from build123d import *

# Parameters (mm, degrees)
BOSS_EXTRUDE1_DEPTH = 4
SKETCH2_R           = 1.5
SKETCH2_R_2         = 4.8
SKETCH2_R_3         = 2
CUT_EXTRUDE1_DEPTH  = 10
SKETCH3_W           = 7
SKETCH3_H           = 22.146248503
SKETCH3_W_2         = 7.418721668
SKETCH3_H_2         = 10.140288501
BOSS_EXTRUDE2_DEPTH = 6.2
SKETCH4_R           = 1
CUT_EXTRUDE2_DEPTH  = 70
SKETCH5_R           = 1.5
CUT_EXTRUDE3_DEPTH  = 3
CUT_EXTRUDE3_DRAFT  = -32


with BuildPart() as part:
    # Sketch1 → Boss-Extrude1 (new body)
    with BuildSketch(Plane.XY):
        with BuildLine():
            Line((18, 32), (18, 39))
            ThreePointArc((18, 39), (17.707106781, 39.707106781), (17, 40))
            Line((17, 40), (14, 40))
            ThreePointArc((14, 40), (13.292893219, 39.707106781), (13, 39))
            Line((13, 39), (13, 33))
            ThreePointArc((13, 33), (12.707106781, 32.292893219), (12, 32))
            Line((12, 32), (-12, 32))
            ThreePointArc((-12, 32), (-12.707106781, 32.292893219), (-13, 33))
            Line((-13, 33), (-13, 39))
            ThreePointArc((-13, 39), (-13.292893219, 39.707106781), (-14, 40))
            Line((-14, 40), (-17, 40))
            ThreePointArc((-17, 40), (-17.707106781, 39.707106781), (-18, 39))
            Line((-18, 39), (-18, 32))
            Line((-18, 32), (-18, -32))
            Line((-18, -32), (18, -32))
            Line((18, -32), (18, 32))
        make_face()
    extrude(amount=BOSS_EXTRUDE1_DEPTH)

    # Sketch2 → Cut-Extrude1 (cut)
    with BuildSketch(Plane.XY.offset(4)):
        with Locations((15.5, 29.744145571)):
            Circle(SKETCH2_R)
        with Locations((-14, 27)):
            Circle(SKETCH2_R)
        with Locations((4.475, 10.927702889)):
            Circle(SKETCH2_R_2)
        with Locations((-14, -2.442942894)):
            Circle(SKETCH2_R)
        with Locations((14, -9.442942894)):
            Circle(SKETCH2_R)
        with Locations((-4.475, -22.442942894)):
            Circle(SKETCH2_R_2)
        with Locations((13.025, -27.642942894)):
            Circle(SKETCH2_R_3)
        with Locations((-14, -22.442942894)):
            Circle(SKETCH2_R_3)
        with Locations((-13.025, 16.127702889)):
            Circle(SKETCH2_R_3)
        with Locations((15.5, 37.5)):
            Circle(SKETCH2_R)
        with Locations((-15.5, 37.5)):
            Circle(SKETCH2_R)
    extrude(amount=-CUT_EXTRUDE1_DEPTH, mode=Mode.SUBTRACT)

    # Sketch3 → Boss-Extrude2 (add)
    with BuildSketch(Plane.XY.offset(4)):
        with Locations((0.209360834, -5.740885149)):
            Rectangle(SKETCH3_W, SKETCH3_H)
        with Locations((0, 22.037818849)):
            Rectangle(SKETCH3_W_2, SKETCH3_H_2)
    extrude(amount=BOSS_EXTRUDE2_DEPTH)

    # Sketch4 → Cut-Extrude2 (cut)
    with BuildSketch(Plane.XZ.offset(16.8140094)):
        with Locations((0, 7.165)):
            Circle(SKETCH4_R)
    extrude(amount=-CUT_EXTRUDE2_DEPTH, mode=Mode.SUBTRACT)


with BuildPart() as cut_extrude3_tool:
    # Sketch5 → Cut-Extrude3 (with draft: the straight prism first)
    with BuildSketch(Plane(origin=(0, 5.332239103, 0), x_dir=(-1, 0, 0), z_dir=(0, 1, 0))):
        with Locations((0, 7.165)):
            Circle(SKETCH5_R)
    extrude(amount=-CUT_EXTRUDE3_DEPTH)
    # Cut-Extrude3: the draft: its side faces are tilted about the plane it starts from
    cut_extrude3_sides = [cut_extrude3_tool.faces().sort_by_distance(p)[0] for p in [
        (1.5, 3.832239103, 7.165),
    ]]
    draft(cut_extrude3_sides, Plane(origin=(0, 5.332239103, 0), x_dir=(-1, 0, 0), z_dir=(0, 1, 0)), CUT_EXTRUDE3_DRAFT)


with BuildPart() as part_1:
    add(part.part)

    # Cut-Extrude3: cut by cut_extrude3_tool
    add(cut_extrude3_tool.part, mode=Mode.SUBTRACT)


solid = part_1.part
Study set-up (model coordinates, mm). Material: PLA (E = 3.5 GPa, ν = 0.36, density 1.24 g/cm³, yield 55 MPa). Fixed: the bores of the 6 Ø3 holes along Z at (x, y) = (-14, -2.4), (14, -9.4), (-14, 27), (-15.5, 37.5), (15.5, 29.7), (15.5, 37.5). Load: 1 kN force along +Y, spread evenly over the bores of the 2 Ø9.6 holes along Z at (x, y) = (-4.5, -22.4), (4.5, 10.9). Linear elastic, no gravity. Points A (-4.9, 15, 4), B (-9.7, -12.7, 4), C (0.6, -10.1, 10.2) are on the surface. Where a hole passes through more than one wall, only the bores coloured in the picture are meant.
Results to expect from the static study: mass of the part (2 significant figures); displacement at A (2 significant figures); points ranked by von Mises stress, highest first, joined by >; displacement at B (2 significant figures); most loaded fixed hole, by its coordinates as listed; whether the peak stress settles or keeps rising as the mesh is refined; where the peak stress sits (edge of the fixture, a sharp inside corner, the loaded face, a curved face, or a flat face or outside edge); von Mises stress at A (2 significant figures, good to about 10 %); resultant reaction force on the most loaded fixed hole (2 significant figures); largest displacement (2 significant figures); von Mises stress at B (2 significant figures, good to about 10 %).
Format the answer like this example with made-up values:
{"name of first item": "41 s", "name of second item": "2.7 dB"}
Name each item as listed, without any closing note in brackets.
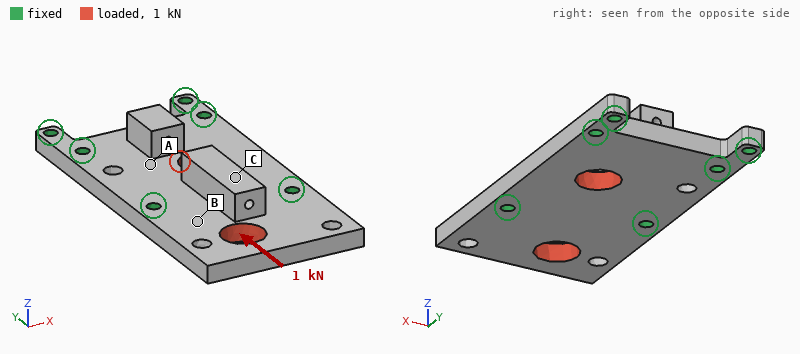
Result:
{"mass of the part": "12 g", "displacement at A": "16 µm", "points ranked by von Mises stress, highest first, joined by >": "B > A > C", "displacement at B": "25 µm", "most loaded fixed hole, by its coordinates as listed": "(-14, -2.4)", "whether the peak stress settles or keeps rising as the mesh is refined": "keeps rising", "where the peak stress sits": "edge of the fixture", "von Mises stress at A": "3.2 MPa", "resultant reaction force on the most loaded fixed hole": "410 N", "largest displacement": "70 µm", "von Mises stress at B": "6.0 MPa"}
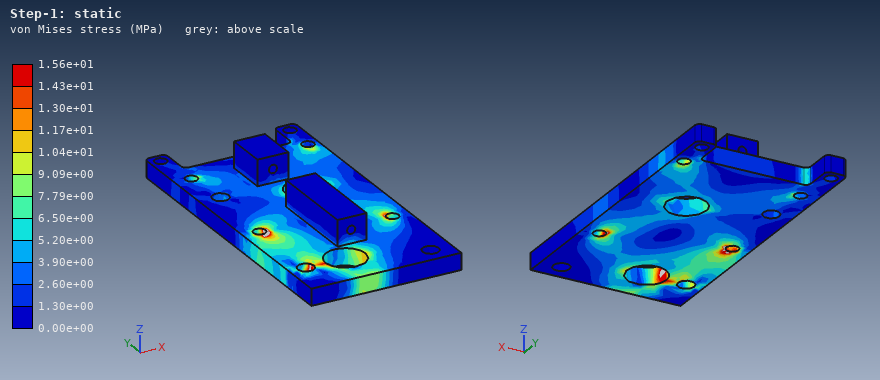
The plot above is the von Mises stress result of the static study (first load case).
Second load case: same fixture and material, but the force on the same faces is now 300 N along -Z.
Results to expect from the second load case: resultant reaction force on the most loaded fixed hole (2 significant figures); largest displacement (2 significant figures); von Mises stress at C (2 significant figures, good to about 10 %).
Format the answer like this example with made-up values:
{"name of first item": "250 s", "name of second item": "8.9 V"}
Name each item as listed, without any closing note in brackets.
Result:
{"resultant reaction force on the most loaded fixed hole": "140 N", "largest displacement": "0.73 mm", "von Mises stress at C": "7.6 MPa"}
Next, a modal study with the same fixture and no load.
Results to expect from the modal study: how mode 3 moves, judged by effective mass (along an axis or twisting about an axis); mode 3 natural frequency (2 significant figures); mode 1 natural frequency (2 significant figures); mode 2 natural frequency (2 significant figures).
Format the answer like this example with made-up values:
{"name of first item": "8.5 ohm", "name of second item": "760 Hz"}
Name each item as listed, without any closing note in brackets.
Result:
{"how mode 3 moves, judged by effective mass": "along Z", "mode 3 natural frequency": "4000 Hz", "mode 1 natural frequency": "1700 Hz", "mode 2 natural frequency": "3100 Hz"}
